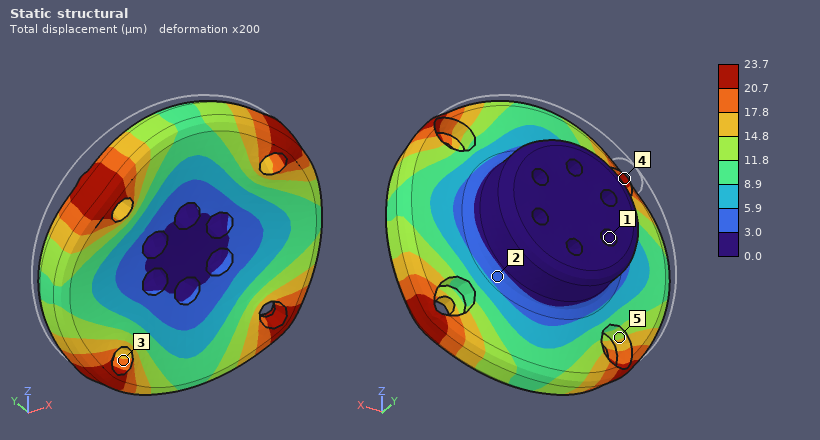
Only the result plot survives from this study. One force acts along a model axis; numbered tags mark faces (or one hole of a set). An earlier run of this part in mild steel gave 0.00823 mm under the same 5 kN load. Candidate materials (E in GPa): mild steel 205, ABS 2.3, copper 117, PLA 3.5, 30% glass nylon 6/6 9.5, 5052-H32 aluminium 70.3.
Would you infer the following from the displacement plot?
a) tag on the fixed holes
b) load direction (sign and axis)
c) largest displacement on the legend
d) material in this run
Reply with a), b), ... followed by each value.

a) 1
b) -Y
c) 23.7 µm
d) 5052-H32 aluminium
